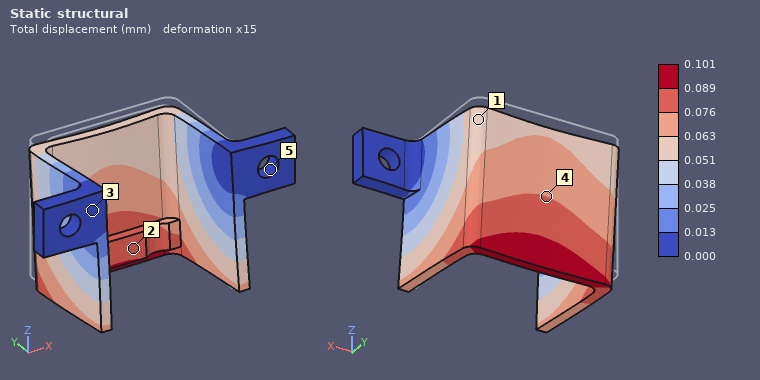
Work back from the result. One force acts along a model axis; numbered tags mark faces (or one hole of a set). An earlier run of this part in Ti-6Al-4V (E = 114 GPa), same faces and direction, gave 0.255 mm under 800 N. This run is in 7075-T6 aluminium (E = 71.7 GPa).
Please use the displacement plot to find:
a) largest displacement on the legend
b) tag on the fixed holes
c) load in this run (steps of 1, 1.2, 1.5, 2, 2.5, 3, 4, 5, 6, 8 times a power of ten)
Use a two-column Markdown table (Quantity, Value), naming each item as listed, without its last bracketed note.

| Quantity | Value |
|---|---|
| largest displacement on the legend | 0.101 mm |
| tag on the fixed holes | 5 |
| load in this run | 200 N |
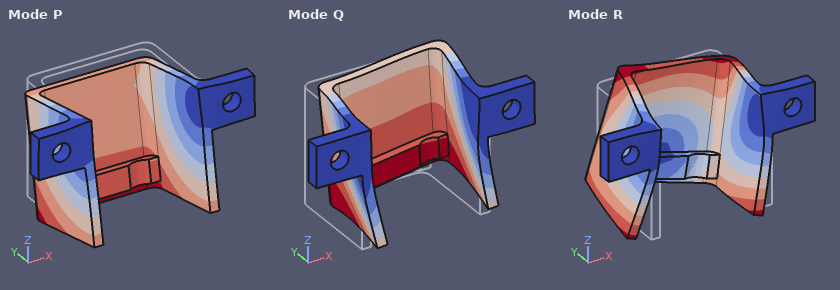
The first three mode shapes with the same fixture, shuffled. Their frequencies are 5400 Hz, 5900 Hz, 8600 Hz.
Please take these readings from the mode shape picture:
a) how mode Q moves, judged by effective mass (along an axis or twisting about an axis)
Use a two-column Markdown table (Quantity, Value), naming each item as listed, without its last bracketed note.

| Quantity | Value |
|---|---|
| how mode Q moves, judged by effective mass | along X |
